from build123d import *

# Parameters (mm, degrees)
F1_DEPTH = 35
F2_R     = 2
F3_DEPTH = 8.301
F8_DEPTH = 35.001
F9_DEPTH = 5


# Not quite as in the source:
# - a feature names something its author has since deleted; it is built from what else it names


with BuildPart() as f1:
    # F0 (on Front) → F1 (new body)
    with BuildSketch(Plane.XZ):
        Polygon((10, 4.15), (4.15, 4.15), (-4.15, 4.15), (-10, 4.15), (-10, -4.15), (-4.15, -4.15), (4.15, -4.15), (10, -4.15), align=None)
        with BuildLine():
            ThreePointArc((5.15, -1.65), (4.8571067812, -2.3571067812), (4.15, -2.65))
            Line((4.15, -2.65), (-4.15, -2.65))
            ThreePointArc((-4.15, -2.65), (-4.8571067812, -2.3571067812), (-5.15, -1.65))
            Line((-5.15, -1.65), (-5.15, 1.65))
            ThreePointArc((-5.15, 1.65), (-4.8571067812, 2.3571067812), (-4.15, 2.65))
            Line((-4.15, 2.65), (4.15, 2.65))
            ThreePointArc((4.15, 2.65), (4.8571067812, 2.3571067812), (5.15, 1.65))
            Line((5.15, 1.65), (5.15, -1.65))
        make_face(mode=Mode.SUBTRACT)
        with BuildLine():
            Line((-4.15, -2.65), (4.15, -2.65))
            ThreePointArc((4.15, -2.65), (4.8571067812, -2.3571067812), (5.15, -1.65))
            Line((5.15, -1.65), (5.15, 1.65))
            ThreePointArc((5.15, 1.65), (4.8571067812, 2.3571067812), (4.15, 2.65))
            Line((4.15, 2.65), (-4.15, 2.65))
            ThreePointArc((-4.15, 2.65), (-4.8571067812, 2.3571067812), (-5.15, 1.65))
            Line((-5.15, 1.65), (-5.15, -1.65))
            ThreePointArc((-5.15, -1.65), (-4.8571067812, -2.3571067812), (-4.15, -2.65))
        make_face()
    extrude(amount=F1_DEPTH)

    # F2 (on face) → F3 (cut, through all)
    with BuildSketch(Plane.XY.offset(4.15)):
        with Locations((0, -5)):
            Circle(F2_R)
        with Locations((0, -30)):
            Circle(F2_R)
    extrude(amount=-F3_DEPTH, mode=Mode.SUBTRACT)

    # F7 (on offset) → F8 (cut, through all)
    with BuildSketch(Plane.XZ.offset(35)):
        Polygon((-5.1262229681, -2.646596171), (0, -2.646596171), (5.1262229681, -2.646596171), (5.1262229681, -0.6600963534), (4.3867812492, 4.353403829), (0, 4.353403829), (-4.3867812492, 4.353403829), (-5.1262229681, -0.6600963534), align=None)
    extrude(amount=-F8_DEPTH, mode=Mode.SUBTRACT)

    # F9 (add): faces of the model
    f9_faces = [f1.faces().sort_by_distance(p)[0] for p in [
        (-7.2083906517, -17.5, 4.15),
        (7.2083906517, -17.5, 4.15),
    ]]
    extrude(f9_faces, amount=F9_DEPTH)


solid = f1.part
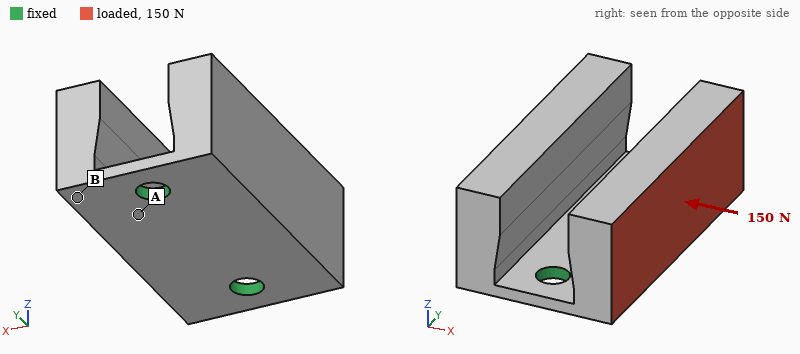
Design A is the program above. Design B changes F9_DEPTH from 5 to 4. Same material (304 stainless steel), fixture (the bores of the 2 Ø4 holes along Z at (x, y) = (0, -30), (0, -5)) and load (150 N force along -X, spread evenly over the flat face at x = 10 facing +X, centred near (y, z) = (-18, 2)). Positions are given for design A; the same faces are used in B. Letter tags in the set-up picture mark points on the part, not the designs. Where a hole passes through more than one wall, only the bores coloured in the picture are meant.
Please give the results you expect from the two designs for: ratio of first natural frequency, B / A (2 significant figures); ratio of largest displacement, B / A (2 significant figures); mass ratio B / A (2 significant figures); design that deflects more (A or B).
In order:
1.1
0.86
0.93
A
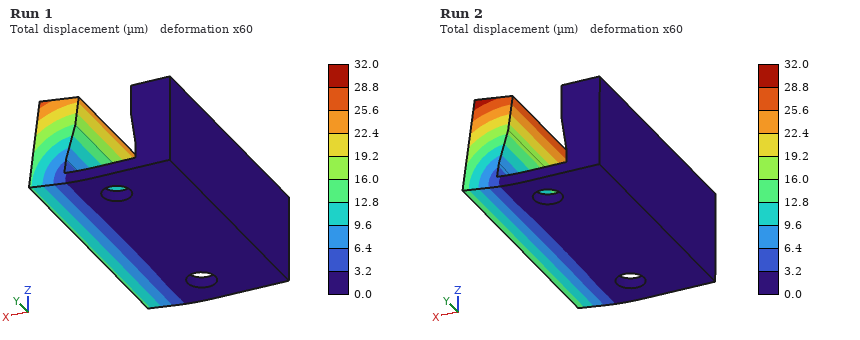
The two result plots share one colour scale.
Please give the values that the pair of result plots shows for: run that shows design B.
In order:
Run 1
